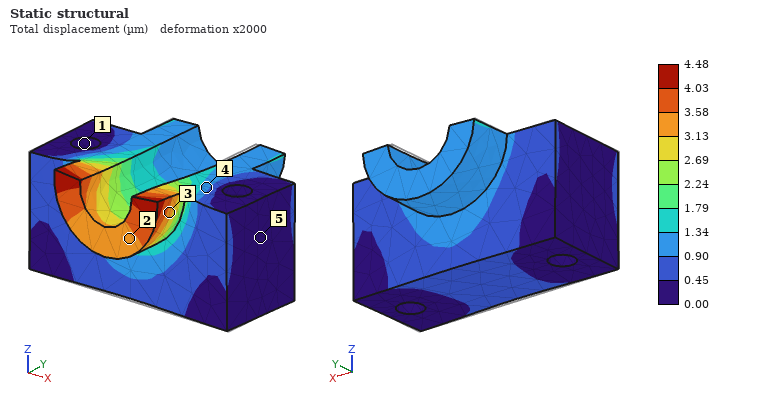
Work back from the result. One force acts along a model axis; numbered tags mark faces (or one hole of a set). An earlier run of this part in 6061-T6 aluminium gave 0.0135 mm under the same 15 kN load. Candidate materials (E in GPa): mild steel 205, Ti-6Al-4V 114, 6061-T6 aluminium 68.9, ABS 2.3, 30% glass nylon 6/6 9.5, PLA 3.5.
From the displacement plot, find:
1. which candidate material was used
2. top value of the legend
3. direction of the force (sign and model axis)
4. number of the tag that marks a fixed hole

mild steel
4.48 µm
+Y
1
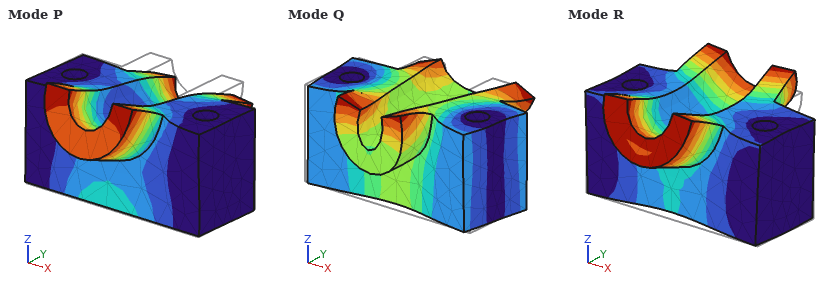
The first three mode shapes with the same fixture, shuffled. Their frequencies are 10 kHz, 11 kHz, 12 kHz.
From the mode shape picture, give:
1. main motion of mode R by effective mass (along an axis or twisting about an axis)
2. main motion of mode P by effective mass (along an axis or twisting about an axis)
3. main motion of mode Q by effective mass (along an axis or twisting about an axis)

along Z
twisting about X
along Y
